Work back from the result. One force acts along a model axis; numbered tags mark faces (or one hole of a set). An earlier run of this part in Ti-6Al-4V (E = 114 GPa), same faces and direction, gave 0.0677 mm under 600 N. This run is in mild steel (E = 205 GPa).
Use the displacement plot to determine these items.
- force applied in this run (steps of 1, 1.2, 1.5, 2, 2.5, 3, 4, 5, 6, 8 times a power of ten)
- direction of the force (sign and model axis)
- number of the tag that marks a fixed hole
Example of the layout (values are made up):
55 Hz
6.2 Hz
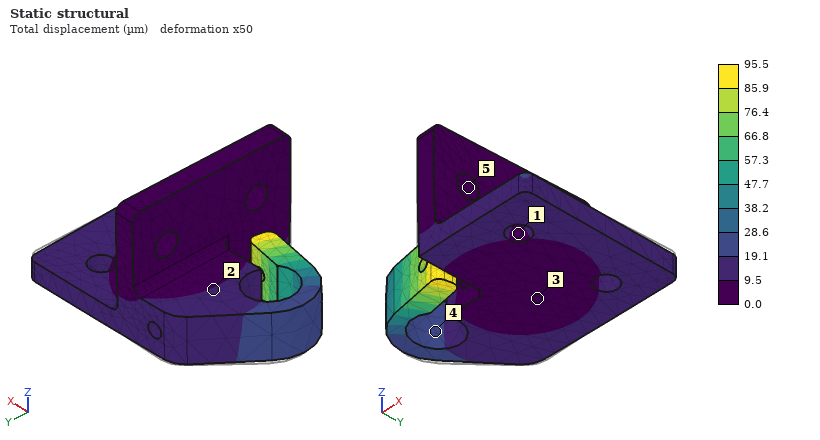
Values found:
1.5 kN
-Y
5
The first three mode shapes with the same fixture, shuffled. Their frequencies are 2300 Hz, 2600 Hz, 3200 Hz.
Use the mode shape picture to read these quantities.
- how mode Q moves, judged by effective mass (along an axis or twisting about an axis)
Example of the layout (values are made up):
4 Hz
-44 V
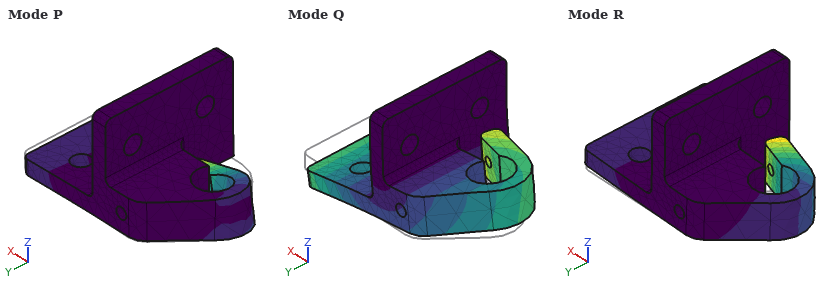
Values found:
along X
